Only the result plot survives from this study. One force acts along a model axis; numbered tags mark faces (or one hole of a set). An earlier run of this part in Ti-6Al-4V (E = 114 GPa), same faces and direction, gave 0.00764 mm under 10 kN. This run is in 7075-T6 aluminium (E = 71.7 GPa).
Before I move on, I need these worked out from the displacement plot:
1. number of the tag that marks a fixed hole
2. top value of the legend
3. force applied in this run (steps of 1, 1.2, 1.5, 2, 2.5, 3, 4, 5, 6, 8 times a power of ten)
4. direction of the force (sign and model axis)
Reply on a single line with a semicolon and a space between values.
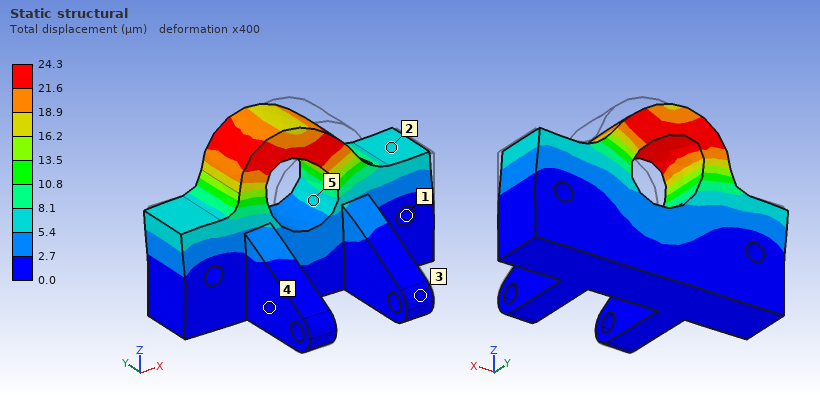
1; 24.3 µm; 20 kN; -X
